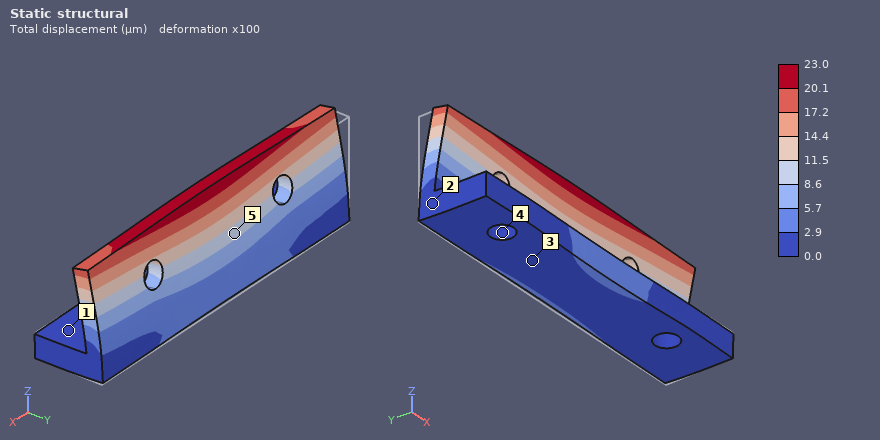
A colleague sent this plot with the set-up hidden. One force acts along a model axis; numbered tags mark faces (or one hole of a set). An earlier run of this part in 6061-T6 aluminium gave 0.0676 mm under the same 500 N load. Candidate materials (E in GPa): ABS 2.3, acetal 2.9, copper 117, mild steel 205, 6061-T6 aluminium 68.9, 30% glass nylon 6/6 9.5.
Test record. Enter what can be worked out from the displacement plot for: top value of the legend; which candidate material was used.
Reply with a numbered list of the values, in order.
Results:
1. 23.0 µm
2. mild steel
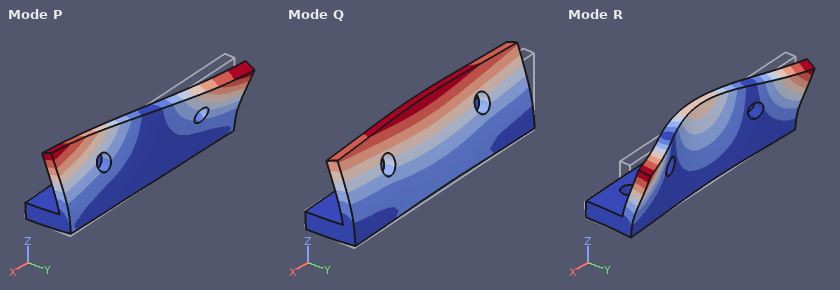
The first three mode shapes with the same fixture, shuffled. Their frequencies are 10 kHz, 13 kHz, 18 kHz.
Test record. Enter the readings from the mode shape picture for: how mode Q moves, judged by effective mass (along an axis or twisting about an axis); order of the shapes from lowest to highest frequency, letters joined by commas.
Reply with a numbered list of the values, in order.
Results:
1. along Y
2. Q, P, R
